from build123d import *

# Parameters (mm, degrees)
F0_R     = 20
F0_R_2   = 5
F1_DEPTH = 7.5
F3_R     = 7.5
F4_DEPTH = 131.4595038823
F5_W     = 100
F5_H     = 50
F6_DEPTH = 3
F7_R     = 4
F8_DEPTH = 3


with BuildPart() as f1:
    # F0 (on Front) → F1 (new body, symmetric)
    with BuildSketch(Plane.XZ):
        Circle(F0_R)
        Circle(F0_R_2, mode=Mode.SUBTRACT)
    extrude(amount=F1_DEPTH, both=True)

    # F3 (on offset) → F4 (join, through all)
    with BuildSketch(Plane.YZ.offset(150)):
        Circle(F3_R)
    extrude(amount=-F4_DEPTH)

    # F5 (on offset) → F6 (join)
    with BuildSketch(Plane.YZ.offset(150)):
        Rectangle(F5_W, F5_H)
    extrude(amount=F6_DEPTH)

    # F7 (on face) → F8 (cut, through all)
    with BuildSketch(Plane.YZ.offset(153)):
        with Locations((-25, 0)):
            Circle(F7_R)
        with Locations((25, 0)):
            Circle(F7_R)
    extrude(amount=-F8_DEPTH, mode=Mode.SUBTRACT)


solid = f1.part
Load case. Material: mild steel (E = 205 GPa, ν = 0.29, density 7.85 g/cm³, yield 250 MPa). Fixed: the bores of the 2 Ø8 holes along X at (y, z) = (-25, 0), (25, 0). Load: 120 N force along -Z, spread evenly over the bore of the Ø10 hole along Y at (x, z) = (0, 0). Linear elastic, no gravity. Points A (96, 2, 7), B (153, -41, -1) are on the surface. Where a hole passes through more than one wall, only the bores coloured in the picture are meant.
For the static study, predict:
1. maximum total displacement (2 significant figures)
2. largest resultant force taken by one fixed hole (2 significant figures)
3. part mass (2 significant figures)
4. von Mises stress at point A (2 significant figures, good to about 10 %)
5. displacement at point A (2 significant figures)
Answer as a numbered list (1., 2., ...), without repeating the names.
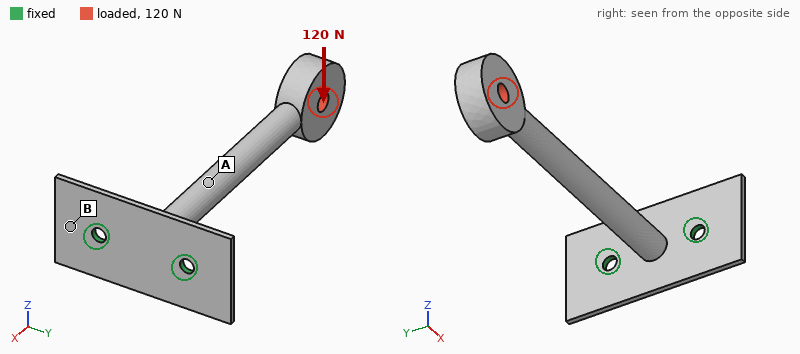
1. 1.1 mm
2. 60 N
3. 430 g
4. 34 MPa
5. 0.30 mm
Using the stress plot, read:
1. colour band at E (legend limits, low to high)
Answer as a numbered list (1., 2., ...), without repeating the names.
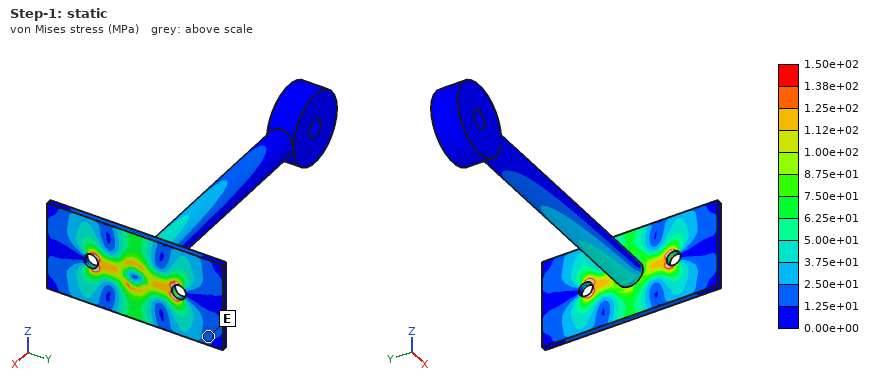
1. 1.25e+01 to 2.50e+01 MPa
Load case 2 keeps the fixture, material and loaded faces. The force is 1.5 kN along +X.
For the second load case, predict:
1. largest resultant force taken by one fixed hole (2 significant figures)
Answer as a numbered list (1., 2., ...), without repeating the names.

1. 780 N
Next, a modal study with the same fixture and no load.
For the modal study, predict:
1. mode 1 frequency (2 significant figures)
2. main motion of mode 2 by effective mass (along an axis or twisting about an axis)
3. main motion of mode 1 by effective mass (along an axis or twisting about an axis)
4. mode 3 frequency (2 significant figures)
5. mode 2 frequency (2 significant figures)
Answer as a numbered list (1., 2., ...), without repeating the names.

1. 130 Hz
2. along Y
3. along Z
4. 1400 Hz
5. 180 Hz
